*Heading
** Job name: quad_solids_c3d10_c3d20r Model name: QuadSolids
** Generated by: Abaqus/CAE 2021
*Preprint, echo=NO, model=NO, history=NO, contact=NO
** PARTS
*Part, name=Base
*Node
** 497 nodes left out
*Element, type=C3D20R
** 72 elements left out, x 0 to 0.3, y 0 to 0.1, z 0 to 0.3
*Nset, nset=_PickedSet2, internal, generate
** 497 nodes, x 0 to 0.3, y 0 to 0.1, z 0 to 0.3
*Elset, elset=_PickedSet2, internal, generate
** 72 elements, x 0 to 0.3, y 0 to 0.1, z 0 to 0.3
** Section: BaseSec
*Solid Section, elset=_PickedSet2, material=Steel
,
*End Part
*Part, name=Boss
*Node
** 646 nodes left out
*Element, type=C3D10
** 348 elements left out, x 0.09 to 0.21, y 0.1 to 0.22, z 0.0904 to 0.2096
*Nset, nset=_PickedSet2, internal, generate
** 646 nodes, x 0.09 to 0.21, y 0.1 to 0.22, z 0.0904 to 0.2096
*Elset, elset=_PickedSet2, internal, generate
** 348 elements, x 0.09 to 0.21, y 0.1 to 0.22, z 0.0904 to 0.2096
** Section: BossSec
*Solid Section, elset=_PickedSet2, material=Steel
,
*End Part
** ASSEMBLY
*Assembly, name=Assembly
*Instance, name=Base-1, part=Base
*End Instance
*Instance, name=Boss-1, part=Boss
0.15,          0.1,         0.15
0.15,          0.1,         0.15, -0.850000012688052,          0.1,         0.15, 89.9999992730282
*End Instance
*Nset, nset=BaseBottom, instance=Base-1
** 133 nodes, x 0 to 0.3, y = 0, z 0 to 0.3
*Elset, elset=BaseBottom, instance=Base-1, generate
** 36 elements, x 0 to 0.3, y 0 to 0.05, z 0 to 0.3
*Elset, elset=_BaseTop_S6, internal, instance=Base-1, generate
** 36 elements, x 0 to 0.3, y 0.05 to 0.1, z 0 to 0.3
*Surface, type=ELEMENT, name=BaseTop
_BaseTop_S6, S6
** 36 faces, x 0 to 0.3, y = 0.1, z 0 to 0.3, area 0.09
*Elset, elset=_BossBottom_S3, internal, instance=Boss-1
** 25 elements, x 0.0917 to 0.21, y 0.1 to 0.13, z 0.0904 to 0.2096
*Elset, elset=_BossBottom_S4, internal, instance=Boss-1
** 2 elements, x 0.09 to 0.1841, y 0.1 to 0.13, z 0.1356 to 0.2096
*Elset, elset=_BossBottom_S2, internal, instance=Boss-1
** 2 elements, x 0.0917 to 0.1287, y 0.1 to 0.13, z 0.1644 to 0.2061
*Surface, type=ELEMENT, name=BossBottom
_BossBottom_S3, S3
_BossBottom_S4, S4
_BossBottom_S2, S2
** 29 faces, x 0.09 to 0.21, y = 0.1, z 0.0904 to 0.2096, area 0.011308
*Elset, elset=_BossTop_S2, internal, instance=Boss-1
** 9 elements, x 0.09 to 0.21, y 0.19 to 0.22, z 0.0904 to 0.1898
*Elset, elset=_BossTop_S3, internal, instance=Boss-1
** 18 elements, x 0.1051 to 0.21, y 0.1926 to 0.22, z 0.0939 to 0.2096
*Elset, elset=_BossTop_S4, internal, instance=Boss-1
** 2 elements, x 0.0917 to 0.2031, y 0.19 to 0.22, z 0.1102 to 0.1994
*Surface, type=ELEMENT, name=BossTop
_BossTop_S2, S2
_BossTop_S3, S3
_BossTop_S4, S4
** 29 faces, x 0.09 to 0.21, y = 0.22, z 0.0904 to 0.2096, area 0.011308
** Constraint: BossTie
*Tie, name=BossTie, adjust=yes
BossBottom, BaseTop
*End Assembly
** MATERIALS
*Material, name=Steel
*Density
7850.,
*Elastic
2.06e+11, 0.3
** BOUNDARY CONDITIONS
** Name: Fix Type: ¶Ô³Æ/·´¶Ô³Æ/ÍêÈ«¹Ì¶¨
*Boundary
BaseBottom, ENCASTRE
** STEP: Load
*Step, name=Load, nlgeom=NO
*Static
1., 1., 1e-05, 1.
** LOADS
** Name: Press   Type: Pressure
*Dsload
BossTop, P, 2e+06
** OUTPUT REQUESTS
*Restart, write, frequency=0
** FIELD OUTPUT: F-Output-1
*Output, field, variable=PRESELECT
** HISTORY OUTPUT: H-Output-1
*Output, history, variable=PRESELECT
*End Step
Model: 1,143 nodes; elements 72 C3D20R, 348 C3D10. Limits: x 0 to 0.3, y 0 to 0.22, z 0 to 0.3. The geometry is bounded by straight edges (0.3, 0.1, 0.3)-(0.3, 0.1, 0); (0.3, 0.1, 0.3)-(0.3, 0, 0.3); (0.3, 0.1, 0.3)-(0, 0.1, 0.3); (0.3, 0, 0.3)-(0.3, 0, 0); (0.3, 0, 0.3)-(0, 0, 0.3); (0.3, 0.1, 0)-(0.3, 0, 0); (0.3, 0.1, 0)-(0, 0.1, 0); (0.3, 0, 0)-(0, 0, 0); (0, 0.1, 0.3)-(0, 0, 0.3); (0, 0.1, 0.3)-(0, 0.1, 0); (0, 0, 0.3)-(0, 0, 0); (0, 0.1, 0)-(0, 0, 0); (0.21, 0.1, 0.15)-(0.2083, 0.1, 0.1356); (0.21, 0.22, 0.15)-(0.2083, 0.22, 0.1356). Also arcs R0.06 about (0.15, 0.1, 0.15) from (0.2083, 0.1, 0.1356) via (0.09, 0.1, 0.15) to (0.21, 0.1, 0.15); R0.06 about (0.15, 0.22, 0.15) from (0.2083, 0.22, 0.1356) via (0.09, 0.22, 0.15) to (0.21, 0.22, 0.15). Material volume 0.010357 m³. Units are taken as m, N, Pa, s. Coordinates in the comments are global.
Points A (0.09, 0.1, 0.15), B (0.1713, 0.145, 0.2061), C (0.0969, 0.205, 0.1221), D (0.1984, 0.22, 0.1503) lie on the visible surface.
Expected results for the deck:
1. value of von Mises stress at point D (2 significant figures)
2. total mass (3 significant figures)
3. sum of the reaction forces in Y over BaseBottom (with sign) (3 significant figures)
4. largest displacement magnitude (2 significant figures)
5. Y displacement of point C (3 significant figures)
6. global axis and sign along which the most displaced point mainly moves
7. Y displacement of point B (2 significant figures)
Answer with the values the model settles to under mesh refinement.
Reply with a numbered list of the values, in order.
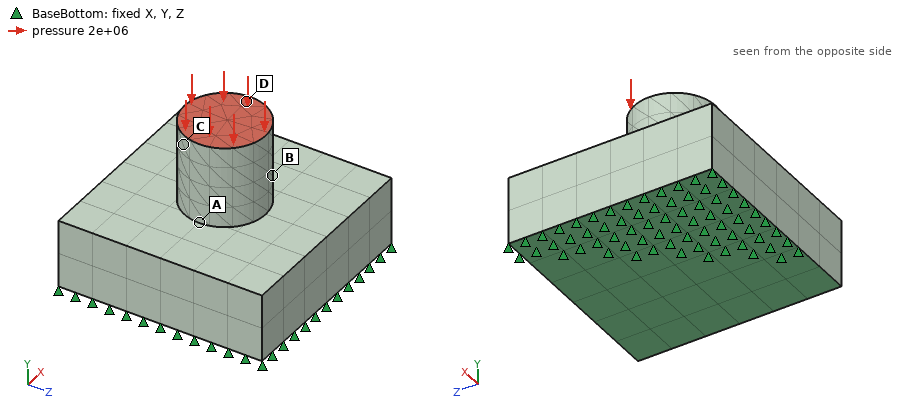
1. 2.0e+06 Pa
2. 81.3 kg
3. 22600 N
4. 1.6e-06 m
5. -1.45e-06 m
6. -Y
7. -8.7e-07 m
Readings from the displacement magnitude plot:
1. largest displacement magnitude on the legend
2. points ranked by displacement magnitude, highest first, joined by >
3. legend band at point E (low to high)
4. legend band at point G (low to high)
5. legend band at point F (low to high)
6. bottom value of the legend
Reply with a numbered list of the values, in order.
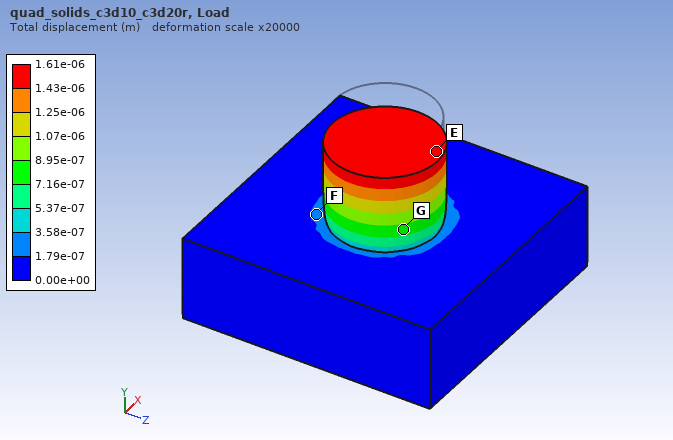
1. 1.61e-06 m
2. E > G > F
3. 1.43e-06 to 1.61e-06 m
4. 7.16e-07 to 8.95e-07 m
5. 1.79e-07 to 3.58e-07 m
6. 0.00e+00 m
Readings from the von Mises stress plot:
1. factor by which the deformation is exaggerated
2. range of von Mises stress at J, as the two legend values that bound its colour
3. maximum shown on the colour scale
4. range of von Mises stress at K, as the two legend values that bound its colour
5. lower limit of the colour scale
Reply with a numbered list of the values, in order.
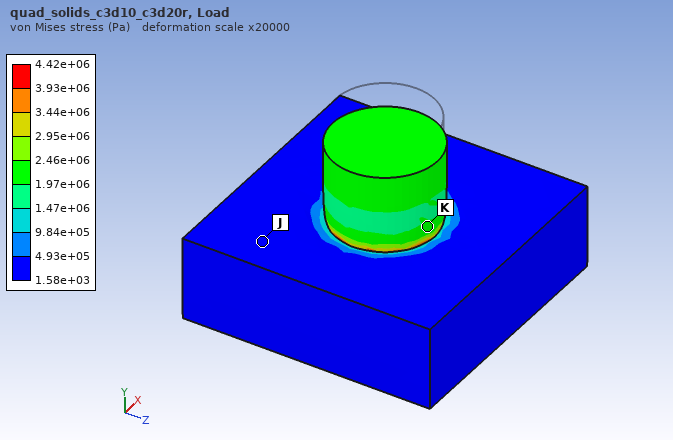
1. 20000
2. 1.58e+03 to 4.93e+05 Pa
3. 4.42e+06 Pa
4. 1.97e+06 to 2.46e+06 Pa
5. 1.58e+03 Pa
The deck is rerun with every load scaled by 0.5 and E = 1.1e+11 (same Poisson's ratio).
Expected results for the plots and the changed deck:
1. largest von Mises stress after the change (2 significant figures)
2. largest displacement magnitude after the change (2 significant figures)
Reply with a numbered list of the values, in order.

1. 2.2e+06 Pa
2. 1.5e-06 m
